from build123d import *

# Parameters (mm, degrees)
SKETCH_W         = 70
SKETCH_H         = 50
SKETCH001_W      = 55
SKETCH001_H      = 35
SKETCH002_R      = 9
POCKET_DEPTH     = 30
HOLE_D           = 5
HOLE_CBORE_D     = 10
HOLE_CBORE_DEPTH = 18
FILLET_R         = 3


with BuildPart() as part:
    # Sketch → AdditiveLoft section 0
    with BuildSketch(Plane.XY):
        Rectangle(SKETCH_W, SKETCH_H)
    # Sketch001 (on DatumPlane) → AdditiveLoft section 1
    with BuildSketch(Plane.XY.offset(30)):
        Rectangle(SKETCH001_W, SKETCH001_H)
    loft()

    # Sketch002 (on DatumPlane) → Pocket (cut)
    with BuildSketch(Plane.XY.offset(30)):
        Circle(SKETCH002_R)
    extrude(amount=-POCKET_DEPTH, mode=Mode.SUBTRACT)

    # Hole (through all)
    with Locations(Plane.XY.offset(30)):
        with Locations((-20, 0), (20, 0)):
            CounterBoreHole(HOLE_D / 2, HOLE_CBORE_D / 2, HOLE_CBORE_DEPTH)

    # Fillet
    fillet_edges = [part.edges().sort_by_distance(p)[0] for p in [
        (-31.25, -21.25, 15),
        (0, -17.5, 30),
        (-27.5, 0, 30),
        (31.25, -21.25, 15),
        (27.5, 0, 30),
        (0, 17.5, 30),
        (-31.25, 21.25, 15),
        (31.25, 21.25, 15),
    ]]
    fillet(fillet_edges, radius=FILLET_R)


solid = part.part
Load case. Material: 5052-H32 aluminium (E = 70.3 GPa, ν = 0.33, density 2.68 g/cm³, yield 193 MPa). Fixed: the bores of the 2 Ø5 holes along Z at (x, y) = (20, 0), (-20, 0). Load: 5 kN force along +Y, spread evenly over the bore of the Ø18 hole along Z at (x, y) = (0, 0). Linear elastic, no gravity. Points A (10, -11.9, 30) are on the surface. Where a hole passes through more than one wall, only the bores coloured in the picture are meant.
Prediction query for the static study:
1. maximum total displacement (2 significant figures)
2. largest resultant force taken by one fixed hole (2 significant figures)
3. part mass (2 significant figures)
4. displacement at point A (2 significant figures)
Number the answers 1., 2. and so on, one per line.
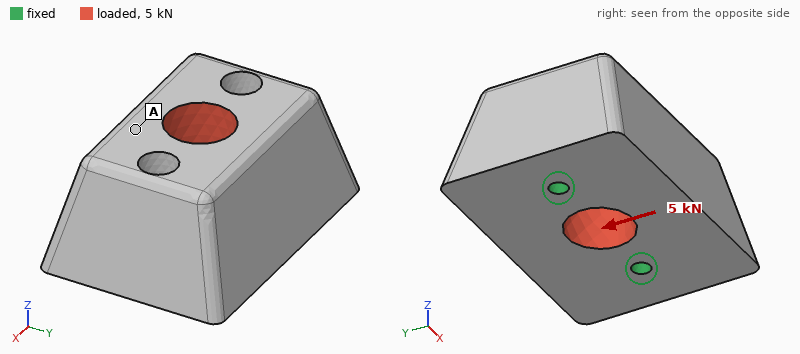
1. 17 µm
2. 2.5 kN
3. 180 g
4. 15 µm
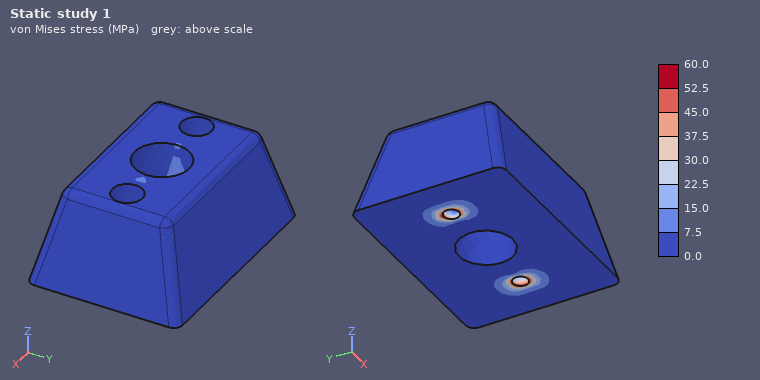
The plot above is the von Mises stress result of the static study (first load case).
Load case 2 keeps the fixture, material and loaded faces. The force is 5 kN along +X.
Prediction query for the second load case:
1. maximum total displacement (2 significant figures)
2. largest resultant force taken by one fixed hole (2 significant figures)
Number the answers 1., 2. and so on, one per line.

1. 4.5 µm
2. 2.7 kN
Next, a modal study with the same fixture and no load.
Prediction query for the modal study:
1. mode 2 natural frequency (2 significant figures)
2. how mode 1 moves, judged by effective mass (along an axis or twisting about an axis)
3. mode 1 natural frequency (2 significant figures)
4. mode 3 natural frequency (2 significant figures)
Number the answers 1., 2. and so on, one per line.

1. 14 kHz
2. along Y
3. 6500 Hz
4. 15 kHz
